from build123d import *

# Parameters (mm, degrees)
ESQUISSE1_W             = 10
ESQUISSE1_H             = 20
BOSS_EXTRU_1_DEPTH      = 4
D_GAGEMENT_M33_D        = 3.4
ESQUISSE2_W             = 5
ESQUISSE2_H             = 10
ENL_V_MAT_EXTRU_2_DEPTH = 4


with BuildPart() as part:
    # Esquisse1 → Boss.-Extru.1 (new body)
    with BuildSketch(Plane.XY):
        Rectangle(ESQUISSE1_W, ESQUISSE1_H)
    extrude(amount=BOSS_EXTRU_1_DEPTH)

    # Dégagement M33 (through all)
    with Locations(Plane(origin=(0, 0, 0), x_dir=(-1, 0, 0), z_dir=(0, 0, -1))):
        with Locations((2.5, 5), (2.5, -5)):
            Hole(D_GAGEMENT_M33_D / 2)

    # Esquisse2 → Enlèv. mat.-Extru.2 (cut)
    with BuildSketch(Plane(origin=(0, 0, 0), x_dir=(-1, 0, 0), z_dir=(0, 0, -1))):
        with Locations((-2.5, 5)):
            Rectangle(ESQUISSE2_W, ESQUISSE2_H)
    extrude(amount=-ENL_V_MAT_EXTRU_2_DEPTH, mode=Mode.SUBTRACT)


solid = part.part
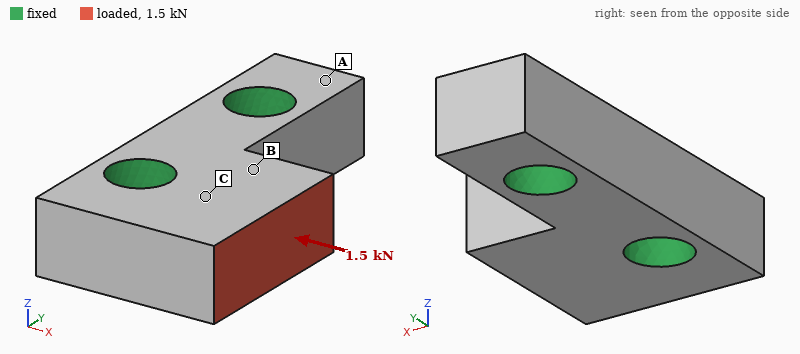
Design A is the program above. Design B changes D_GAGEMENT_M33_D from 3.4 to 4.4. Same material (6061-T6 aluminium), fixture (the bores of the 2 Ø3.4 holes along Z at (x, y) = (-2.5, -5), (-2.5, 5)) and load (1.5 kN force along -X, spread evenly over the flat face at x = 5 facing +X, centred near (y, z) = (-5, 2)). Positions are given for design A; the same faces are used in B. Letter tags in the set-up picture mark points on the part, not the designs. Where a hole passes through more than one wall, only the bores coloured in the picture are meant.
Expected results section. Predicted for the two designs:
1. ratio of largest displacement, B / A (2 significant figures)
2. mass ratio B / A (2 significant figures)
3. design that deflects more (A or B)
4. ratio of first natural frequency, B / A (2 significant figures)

0.83
0.91
A
1.2
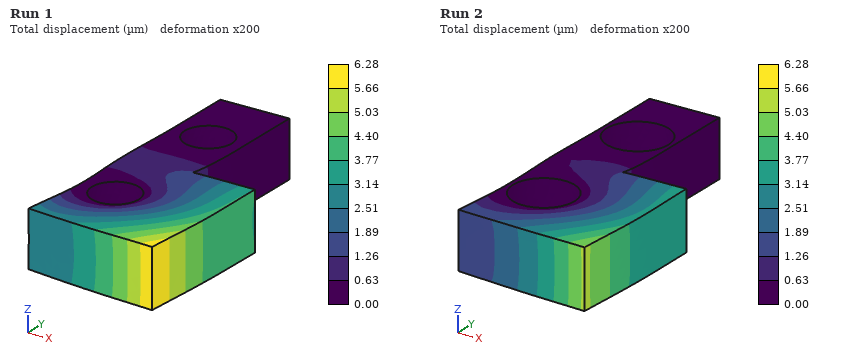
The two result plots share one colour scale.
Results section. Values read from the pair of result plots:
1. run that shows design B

Run 2
